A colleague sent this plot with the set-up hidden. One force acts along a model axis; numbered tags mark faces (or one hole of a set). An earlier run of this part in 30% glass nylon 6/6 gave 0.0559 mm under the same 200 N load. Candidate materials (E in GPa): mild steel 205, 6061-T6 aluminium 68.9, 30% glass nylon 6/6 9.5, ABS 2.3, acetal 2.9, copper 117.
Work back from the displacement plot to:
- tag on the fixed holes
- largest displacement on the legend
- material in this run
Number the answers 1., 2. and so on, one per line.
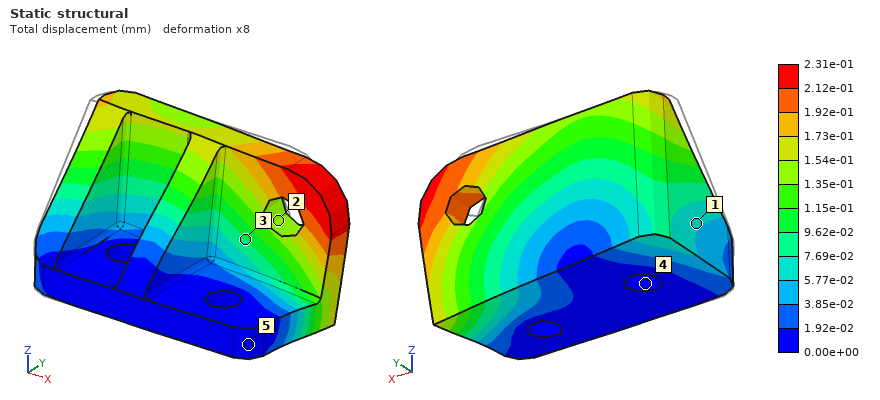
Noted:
1. 4
2. 2.31e-01 mm
3. ABS
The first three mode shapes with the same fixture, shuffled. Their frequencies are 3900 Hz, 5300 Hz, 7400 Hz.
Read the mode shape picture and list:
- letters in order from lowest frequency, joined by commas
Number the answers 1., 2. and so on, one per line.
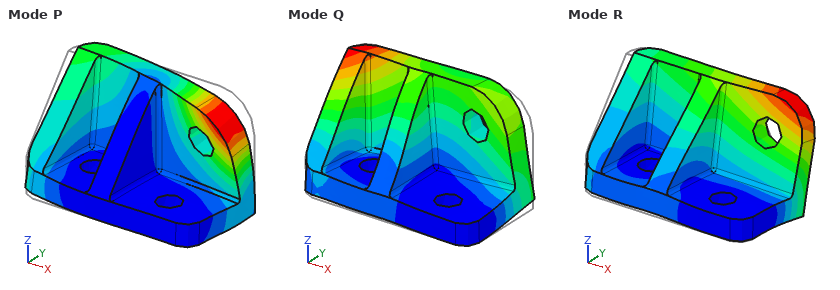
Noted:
1. R, Q, P
